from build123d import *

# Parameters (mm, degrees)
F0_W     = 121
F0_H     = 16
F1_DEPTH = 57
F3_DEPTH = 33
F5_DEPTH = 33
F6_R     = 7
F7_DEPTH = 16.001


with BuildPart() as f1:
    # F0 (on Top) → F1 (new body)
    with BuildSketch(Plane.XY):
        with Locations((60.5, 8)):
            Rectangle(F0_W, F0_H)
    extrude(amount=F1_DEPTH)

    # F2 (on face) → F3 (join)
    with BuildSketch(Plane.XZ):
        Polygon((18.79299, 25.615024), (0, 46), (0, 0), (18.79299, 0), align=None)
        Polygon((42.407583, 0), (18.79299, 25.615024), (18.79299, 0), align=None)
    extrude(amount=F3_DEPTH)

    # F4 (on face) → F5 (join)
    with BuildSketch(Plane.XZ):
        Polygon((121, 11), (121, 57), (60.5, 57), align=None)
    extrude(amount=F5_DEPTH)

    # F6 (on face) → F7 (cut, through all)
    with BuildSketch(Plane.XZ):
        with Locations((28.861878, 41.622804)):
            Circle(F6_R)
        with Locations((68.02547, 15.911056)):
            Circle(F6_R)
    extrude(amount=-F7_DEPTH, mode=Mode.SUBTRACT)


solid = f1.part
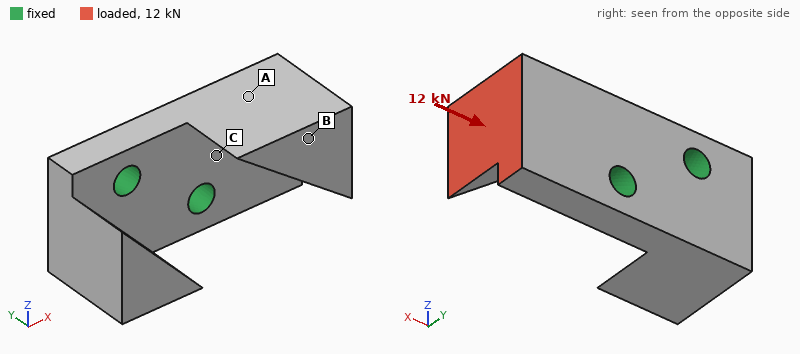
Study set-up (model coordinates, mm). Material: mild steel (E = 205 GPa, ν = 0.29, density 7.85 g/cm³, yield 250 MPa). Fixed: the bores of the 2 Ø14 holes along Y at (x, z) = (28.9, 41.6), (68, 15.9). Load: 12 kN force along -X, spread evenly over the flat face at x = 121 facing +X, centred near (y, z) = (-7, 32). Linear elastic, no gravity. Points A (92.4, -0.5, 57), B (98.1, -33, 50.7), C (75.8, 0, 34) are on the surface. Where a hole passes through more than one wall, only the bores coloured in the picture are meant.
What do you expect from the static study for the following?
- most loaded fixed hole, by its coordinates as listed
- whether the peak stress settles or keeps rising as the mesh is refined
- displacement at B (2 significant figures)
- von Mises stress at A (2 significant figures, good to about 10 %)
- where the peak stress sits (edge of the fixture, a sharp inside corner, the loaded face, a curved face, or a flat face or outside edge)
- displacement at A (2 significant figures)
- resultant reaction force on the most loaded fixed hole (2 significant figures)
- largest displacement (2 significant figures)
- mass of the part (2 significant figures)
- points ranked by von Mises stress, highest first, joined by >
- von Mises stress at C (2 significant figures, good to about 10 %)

(68, 15.9)
keeps rising
57 µm
24 MPa
edge of the fixture
28 µm
7.8 kN
76 µm
1.4 kg
C > A > B
65 MPa
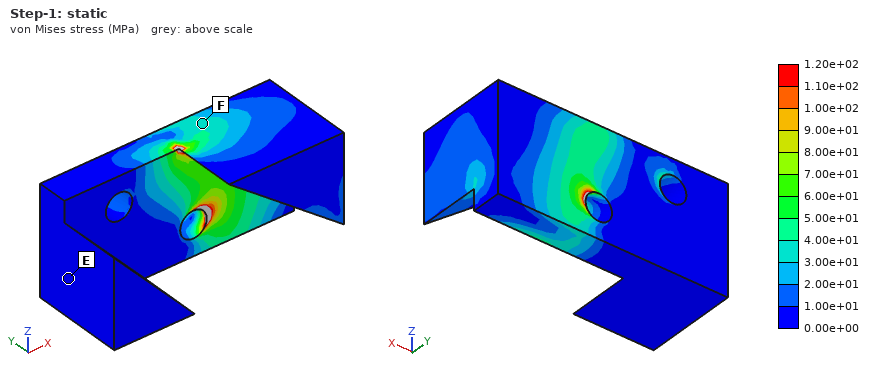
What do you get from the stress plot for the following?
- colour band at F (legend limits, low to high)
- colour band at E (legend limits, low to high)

3.00e+01 to 4.00e+01 MPa
0.00e+00 to 1.00e+01 MPa
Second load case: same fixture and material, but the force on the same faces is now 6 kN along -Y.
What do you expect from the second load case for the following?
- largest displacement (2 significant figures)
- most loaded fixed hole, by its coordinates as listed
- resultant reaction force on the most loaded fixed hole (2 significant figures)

0.11 mm
(68, 15.9)
8.2 kN
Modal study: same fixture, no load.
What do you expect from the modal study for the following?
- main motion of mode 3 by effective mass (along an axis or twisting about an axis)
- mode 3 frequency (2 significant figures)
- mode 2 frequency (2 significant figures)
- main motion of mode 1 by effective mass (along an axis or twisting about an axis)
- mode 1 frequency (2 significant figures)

along Z
3900 Hz
3500 Hz
along Y
2100 Hz
